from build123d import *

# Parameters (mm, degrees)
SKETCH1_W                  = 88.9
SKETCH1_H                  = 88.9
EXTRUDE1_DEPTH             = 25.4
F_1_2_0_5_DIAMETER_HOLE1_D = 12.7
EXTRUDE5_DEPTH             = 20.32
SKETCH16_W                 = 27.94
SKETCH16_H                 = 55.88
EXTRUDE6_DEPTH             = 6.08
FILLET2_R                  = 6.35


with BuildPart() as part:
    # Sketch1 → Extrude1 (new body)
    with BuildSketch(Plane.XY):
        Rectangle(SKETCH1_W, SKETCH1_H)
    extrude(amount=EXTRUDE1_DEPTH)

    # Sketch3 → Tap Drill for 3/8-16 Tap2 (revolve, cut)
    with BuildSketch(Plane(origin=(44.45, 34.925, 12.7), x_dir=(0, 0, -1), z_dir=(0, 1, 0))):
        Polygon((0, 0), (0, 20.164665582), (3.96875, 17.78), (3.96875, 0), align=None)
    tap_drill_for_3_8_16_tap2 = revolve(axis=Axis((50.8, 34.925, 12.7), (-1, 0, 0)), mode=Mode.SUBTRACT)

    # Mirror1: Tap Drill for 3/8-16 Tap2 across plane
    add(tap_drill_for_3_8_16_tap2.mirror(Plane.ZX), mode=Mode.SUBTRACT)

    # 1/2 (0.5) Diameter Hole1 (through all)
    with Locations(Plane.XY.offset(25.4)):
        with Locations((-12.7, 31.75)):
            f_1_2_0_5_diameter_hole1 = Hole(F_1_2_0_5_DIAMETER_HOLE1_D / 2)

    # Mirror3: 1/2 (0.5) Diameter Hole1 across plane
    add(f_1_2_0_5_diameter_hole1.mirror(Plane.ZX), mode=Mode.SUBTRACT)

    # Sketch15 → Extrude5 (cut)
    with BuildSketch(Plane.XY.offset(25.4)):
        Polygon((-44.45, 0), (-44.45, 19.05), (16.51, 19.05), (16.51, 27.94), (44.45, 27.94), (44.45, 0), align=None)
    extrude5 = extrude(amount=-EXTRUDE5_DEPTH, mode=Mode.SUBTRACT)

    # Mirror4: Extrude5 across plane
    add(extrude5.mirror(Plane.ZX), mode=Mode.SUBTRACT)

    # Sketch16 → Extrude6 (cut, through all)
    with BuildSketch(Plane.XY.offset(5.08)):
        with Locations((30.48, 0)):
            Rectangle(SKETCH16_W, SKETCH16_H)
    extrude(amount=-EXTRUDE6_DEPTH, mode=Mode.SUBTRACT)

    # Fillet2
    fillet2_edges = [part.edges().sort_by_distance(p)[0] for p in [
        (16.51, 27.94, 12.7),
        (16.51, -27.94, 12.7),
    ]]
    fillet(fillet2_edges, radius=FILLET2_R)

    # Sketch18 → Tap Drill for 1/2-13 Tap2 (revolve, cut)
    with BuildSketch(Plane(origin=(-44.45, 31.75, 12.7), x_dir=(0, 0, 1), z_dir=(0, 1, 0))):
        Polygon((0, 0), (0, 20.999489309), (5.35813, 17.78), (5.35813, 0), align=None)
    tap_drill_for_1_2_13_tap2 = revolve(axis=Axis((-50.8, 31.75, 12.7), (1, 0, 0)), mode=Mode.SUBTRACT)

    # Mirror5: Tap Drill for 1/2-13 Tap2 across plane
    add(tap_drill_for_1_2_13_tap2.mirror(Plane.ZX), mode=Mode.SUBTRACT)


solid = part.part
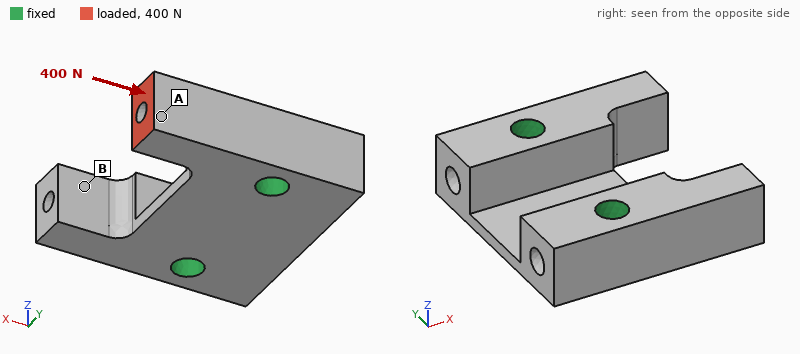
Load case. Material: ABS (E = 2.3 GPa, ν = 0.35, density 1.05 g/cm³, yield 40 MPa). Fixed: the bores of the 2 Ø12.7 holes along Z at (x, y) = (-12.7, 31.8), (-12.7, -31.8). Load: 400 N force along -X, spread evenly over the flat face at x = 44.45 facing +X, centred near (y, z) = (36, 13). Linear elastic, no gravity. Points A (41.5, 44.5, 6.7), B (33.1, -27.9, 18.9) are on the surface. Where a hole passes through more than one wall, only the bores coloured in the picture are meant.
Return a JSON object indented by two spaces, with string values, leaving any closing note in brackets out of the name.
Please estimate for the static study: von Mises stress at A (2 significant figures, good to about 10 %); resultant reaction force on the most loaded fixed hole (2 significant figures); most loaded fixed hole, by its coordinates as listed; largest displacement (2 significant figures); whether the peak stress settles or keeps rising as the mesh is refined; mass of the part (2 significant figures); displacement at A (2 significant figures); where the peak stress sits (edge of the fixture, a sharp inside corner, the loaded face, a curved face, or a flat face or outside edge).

{
  "von Mises stress at A": "1.1 MPa",
  "resultant reaction force on the most loaded fixed hole": "410 N",
  "most loaded fixed hole, by its coordinates as listed": "(-12.7, 31.8)",
  "largest displacement": "40 µm",
  "whether the peak stress settles or keeps rising as the mesh is refined": "keeps rising",
  "mass of the part": "110 g",
  "displacement at A": "37 µm",
  "where the peak stress sits": "edge of the fixture"
}
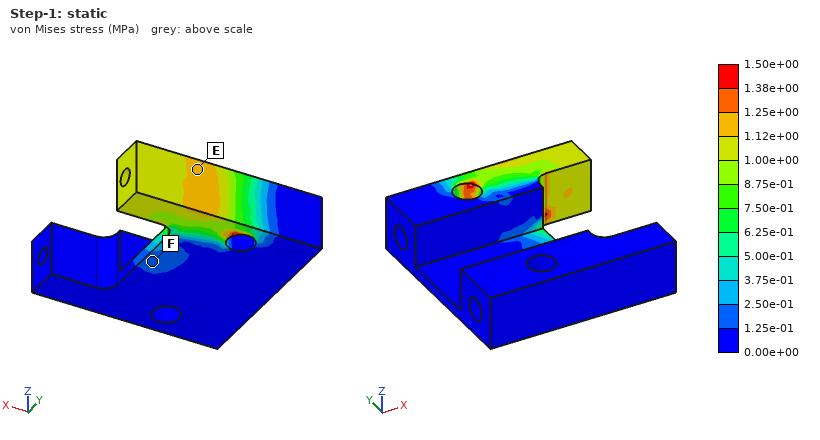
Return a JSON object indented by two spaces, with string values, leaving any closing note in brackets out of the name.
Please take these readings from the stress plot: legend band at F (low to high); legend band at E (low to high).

{
  "legend band at F": "1.25e-01 to 2.50e-01 MPa",
  "legend band at E": "1.12e+00 to 1.25e+00 MPa"
}
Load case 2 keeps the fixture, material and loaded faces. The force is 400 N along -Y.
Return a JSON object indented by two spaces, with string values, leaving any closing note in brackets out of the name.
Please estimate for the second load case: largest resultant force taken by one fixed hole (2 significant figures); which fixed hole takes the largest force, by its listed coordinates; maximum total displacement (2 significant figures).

{
  "largest resultant force taken by one fixed hole": "300 N",
  "which fixed hole takes the largest force, by its listed coordinates": "(-12.7, 31.8)",
  "maximum total displacement": "0.46 mm"
}
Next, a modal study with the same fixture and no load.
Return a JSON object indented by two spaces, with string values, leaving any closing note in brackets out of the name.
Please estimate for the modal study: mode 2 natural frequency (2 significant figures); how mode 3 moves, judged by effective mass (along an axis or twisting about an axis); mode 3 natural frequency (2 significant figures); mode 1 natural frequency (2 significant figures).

{
  "mode 2 natural frequency": "2100 Hz",
  "how mode 3 moves, judged by effective mass": "along Z",
  "mode 3 natural frequency": "2300 Hz",
  "mode 1 natural frequency": "2100 Hz"
}
